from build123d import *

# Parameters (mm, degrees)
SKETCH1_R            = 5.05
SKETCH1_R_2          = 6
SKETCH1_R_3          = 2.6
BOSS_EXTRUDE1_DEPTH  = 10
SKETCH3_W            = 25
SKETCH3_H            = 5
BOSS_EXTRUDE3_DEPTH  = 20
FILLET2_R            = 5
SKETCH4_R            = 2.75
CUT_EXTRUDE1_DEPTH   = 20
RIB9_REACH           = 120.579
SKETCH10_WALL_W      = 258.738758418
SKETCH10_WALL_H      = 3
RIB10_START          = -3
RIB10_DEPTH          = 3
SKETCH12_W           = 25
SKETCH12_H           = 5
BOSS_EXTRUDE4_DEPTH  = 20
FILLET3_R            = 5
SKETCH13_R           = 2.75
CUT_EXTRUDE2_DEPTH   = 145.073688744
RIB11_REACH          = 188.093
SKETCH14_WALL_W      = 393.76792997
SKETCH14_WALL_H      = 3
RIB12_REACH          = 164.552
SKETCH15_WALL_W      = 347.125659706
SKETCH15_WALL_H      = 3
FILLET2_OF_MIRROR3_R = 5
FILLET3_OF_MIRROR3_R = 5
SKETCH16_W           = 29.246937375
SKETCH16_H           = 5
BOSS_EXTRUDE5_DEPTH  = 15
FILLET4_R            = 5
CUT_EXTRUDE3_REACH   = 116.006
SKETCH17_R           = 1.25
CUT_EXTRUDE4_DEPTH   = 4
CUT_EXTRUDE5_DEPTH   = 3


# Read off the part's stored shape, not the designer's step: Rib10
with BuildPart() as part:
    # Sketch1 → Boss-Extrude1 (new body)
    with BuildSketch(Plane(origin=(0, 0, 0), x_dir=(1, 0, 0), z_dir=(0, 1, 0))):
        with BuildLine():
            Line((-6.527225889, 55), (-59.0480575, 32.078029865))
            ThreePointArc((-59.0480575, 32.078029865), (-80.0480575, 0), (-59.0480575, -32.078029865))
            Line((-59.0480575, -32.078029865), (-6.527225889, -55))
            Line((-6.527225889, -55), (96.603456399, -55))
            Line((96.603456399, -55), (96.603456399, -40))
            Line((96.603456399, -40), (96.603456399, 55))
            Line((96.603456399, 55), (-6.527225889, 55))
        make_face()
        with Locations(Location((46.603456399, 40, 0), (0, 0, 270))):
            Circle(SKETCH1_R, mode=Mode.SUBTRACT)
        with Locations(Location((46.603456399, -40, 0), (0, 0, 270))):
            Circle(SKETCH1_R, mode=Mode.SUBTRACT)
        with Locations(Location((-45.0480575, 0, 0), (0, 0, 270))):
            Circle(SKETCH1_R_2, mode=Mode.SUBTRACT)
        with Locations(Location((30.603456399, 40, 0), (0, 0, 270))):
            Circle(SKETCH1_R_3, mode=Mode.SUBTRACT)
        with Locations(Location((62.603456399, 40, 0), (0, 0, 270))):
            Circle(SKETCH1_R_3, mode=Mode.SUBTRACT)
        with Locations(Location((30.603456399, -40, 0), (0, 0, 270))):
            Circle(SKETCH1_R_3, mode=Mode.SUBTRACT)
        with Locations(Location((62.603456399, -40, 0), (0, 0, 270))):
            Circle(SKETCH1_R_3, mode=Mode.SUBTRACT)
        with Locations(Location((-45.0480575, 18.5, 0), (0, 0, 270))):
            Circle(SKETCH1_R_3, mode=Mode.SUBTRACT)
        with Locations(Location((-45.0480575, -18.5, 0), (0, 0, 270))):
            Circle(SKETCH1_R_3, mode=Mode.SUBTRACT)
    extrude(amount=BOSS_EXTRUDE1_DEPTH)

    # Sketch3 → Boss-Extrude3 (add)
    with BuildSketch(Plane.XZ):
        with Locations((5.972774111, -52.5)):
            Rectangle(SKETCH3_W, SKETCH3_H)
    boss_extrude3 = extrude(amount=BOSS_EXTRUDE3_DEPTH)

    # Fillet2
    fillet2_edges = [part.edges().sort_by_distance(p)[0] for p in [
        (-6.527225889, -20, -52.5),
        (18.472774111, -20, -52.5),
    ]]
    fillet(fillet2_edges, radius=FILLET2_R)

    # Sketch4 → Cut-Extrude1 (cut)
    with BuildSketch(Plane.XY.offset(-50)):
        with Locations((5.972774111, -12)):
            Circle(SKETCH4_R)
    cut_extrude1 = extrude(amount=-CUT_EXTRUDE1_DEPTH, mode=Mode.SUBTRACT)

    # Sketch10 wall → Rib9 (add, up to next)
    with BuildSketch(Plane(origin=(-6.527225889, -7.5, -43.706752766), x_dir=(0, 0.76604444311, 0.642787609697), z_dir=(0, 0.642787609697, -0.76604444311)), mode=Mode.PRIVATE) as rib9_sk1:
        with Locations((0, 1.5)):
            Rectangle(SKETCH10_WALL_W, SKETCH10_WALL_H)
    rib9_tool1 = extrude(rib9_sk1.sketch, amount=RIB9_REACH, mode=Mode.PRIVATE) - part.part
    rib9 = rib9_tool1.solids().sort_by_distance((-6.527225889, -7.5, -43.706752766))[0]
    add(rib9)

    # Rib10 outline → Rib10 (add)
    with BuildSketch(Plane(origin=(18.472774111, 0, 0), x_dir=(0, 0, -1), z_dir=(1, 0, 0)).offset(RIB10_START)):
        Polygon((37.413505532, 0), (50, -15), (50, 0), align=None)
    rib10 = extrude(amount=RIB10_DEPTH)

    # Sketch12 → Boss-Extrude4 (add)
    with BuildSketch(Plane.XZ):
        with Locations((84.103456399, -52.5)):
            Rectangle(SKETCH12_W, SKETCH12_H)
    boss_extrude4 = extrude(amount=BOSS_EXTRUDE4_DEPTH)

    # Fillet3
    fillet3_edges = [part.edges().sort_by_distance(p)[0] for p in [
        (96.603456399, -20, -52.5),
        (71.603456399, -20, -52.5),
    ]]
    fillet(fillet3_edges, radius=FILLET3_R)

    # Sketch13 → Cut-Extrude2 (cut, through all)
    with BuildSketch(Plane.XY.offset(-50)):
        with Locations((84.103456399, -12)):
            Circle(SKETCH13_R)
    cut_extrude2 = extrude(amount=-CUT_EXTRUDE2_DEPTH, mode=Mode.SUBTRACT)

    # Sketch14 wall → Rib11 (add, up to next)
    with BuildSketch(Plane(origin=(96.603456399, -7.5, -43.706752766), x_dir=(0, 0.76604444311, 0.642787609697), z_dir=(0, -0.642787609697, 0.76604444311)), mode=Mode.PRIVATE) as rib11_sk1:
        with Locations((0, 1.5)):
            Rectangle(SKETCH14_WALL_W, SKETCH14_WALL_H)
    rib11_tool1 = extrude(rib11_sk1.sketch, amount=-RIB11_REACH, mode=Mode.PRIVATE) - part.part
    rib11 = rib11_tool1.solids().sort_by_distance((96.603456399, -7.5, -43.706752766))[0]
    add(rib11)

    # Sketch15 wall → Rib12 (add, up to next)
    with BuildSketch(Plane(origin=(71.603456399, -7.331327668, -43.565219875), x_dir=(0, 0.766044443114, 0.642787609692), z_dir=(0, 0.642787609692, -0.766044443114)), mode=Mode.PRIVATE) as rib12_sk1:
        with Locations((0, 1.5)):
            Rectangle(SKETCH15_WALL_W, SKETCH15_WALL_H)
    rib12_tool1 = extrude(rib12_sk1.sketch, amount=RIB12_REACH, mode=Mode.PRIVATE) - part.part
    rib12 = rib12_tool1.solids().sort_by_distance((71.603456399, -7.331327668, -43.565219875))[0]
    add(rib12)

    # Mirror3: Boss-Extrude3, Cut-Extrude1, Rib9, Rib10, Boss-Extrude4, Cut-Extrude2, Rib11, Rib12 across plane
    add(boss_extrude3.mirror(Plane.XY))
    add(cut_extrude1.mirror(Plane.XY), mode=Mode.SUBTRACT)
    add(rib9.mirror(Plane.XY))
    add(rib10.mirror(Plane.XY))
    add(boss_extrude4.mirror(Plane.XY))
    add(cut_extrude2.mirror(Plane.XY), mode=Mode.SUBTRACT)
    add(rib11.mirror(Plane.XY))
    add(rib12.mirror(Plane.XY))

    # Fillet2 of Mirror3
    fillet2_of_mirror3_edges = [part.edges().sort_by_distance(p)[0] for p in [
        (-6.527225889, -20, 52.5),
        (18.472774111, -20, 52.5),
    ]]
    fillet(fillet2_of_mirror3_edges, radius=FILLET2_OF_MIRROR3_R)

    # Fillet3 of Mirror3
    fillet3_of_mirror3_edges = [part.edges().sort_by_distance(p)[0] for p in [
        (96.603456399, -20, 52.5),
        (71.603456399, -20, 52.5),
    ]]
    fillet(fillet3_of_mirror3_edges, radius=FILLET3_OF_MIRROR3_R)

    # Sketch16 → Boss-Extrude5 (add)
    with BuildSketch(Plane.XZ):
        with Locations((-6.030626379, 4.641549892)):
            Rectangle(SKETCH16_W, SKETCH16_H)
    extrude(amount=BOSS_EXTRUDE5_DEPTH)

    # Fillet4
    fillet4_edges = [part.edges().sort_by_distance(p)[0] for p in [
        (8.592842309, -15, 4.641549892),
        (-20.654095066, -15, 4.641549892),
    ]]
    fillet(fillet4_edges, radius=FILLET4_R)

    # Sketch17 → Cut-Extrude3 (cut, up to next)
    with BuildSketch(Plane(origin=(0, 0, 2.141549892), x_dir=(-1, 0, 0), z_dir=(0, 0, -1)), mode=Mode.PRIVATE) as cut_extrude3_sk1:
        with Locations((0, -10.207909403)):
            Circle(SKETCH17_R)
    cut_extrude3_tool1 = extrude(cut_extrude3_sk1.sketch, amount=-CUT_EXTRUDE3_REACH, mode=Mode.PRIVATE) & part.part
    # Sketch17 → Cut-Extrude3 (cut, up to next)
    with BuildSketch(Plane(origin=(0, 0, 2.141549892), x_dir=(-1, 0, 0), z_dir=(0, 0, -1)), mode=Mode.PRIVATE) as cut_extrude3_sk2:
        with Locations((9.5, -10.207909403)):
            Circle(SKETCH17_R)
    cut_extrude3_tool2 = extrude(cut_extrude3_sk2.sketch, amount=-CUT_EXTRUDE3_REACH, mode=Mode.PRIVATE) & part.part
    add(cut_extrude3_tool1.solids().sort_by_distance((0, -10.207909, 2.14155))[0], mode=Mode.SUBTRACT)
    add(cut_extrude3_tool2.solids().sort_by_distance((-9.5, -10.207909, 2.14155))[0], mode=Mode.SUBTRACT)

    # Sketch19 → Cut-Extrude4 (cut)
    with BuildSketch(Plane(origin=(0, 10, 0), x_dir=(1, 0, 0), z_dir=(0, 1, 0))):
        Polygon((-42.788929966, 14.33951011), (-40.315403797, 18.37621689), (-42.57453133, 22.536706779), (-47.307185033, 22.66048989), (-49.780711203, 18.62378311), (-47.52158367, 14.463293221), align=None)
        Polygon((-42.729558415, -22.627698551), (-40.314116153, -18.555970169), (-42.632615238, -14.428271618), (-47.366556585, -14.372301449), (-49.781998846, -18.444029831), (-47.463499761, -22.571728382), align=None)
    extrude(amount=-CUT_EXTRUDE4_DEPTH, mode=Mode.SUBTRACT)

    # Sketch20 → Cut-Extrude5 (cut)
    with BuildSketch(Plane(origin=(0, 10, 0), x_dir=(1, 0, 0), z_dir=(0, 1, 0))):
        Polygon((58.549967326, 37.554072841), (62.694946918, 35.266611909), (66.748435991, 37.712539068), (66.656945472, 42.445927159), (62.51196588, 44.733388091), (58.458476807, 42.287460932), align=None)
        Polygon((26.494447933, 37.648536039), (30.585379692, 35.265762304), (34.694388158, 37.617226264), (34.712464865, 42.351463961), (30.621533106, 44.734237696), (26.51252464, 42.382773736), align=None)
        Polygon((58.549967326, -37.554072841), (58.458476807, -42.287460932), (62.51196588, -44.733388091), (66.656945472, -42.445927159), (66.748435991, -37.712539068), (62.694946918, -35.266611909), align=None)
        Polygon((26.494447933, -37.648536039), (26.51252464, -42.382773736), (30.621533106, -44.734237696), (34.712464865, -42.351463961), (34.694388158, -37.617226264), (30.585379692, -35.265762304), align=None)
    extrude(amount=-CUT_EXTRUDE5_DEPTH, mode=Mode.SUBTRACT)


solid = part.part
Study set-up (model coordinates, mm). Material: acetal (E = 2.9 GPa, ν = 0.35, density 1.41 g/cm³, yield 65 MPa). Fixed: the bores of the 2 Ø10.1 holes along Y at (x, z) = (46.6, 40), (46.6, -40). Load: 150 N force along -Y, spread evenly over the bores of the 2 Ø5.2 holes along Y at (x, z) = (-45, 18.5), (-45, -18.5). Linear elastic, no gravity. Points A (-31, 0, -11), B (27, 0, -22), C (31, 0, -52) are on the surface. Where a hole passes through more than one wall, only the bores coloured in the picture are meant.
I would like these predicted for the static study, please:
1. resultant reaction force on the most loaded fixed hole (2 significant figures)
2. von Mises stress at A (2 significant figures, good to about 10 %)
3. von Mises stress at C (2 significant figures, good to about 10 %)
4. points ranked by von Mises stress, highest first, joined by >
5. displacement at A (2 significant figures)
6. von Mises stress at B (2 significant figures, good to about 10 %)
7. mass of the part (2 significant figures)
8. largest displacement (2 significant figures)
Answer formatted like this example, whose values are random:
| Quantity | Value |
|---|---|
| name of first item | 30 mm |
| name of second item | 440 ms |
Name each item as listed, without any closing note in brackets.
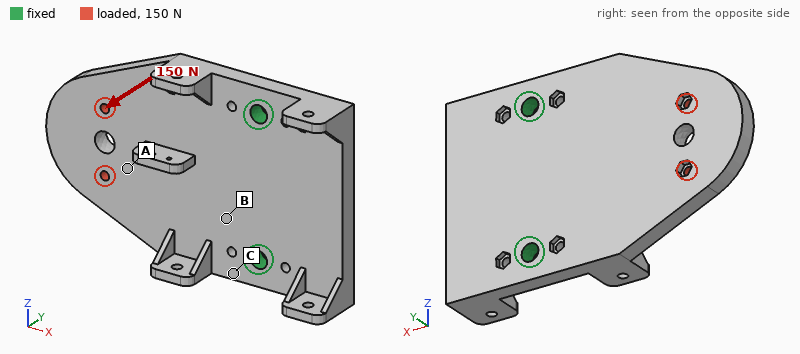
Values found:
| Quantity | Value |
|---|---|
| resultant reaction force on the most loaded fixed hole | 75 N |
| von Mises stress at A | 1.9 MPa |
| von Mises stress at C | 8.4 MPa |
| points ranked by von Mises stress, highest first, joined by > | C > B > A |
| displacement at A | 1.3 mm |
| von Mises stress at B | 5.3 MPa |
| mass of the part | 250 g |
| largest displacement | 2.5 mm |
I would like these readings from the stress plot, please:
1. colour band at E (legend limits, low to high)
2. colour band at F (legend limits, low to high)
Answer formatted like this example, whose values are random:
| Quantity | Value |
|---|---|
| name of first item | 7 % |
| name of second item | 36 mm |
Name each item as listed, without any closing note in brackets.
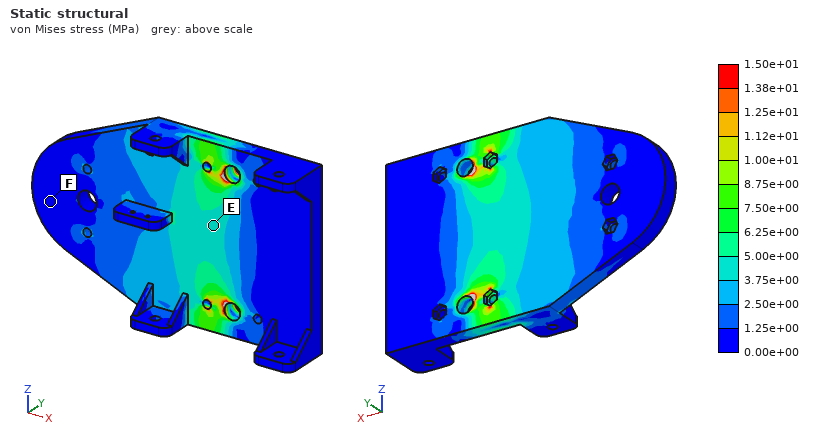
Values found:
| Quantity | Value |
|---|---|
| colour band at E | 3.75e+00 to 5.00e+00 MPa |
| colour band at F | 0.00e+00 to 1.25e+00 MPa |
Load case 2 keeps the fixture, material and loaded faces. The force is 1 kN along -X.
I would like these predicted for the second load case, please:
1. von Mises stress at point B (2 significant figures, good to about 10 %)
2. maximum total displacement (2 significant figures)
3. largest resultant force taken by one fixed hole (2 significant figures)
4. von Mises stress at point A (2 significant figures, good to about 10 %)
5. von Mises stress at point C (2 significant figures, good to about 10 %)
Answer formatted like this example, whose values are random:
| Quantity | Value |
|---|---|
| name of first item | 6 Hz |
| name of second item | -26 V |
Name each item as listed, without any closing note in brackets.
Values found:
| Quantity | Value |
|---|---|
| von Mises stress at point B | 1.8 MPa |
| maximum total displacement | 0.58 mm |
| largest resultant force taken by one fixed hole | 500 N |
| von Mises stress at point A | 2.7 MPa |
| von Mises stress at point C | 2.2 MPa |
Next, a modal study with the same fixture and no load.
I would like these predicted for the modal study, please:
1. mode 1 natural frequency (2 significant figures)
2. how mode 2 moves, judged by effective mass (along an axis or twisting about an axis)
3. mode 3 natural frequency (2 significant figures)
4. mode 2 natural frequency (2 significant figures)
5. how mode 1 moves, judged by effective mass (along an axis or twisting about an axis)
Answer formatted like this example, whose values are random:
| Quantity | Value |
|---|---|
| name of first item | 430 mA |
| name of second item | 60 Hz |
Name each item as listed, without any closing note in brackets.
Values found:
| Quantity | Value |
|---|---|
| mode 1 natural frequency | 180 Hz |
| how mode 2 moves, judged by effective mass | twisting about X |
| mode 3 natural frequency | 720 Hz |
| mode 2 natural frequency | 600 Hz |
| how mode 1 moves, judged by effective mass | along Y |
